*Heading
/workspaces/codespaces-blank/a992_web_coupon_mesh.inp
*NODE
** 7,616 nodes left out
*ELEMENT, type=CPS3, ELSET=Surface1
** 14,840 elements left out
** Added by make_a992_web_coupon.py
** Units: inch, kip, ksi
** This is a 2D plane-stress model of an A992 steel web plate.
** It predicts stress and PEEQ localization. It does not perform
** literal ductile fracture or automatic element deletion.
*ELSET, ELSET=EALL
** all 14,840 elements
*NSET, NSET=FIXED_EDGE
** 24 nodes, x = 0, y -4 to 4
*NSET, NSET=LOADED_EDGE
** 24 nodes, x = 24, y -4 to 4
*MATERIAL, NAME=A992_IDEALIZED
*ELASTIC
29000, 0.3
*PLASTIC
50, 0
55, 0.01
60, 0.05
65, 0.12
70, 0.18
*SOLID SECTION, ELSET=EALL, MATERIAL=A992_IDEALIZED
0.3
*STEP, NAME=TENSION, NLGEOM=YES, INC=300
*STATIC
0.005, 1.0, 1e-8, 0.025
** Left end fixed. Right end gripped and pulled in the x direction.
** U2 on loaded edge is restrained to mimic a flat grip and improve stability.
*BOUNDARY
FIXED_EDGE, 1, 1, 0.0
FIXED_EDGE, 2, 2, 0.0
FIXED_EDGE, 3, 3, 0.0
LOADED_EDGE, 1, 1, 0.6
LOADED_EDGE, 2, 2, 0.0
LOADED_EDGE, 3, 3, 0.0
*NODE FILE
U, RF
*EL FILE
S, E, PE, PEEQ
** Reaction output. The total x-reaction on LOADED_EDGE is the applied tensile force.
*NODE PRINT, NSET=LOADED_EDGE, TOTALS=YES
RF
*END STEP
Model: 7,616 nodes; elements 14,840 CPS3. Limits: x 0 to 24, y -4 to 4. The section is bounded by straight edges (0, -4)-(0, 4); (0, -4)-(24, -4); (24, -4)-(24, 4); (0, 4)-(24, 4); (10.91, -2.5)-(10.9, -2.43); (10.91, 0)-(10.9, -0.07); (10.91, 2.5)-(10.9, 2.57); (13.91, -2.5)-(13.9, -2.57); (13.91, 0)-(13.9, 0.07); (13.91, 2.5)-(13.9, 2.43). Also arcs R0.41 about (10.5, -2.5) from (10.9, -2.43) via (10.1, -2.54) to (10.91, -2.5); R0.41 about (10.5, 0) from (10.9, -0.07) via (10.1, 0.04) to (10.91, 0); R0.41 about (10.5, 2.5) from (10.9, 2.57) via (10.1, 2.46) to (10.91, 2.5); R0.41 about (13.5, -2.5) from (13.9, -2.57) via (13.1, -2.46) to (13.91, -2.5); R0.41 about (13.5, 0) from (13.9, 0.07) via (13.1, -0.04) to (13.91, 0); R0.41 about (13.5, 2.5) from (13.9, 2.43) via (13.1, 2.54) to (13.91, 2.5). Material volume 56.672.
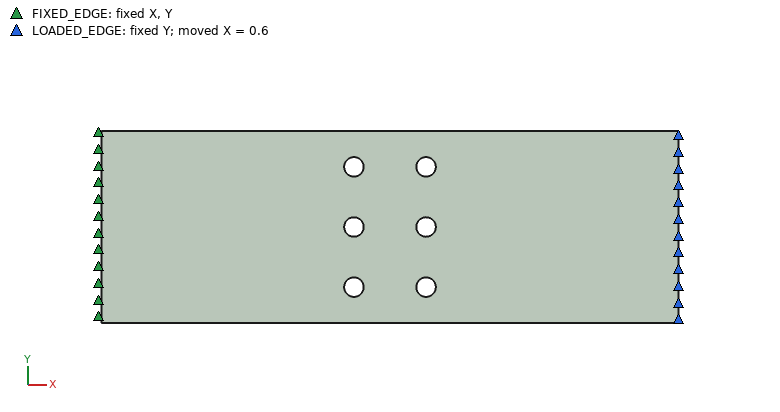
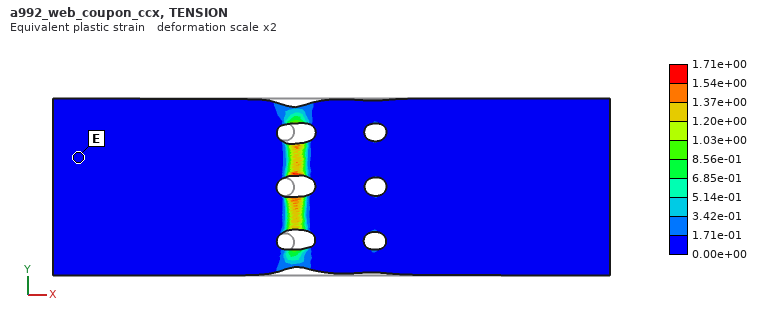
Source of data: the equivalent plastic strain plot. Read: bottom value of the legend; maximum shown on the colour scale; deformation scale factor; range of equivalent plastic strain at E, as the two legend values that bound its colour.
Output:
0.00e+00
1.71e+00
2
0.00e+00 to 1.71e-01
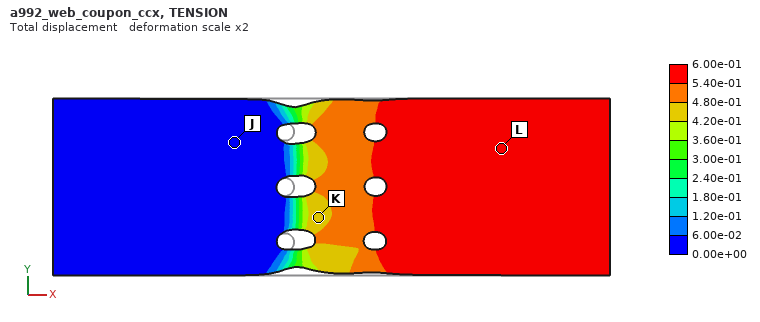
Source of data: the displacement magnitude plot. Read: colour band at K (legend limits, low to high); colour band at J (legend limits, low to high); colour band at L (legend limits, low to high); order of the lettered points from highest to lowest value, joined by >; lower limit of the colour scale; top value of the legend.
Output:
4.20e-01 to 4.80e-01
0.00e+00 to 6.00e-02
5.40e-01 to 6.00e-01
L > K > J
0.00e+00
6.00e-01
